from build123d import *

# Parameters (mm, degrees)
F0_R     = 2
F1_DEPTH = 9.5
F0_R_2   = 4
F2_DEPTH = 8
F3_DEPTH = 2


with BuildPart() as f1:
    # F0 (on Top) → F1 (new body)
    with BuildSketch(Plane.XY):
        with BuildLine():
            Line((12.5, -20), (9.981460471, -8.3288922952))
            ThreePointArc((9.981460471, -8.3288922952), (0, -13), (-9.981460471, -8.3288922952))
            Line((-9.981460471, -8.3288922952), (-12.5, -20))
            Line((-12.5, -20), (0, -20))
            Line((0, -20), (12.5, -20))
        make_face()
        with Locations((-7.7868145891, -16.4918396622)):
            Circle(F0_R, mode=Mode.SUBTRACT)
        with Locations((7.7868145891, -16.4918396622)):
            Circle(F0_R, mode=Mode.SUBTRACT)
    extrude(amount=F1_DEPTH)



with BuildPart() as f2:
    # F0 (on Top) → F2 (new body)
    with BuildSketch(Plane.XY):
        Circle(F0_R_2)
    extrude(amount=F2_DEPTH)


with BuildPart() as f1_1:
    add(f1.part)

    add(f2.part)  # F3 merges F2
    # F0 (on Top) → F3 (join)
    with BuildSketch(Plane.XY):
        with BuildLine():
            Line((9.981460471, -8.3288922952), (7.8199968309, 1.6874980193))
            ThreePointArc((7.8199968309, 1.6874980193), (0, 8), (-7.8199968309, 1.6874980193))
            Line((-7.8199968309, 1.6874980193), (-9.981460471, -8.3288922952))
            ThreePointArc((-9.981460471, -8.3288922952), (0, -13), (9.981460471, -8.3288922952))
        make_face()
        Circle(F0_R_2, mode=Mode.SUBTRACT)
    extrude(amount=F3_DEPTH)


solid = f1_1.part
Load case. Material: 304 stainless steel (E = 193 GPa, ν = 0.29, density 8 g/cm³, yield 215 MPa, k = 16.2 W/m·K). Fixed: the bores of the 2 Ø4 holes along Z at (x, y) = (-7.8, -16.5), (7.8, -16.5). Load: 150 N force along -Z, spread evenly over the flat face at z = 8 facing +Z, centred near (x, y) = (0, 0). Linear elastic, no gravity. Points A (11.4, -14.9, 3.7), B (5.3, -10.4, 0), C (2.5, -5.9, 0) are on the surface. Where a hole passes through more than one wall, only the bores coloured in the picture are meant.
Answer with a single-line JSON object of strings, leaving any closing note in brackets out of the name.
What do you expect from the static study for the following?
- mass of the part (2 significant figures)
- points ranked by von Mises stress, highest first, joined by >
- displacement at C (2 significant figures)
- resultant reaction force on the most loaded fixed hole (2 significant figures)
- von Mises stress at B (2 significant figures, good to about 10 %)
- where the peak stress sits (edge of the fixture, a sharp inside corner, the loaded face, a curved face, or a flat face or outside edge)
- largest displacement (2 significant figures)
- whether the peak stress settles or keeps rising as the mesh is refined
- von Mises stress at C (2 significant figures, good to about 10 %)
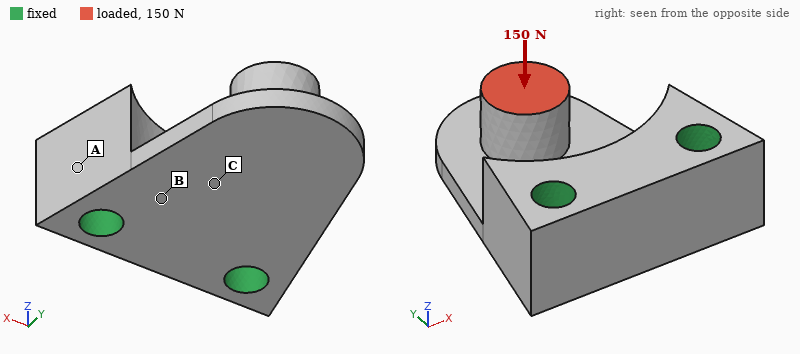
{"mass of the part": "21 g", "points ranked by von Mises stress, highest first, joined by >": "B > C > A", "displacement at C": "13 µm", "resultant reaction force on the most loaded fixed hole": "76 N", "von Mises stress at B": "88 MPa", "where the peak stress sits": "a sharp inside corner", "largest displacement": "67 µm", "whether the peak stress settles or keeps rising as the mesh is refined": "keeps rising", "von Mises stress at C": "67 MPa"}
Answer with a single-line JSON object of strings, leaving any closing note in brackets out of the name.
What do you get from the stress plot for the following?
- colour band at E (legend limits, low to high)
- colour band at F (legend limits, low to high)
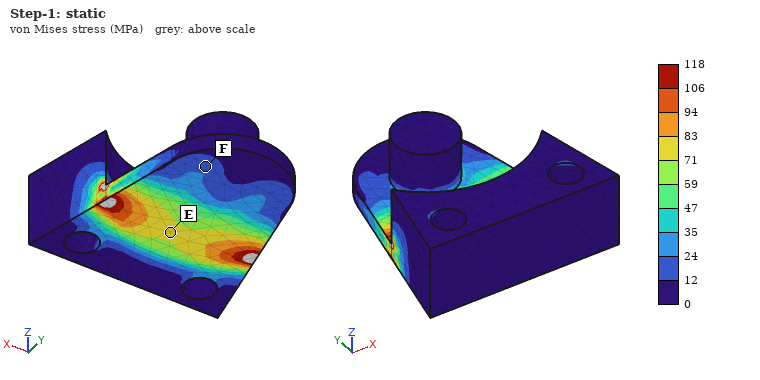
{"colour band at E": "71 to 83 MPa", "colour band at F": "12 to 24 MPa"}
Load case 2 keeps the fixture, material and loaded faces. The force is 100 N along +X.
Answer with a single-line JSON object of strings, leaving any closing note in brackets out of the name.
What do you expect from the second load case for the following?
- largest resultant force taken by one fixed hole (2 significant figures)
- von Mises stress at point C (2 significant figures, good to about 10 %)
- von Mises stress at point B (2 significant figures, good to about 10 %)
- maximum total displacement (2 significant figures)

{"largest resultant force taken by one fixed hole": "110 N", "von Mises stress at point C": "25 MPa", "von Mises stress at point B": "19 MPa", "maximum total displacement": "8.9 µm"}
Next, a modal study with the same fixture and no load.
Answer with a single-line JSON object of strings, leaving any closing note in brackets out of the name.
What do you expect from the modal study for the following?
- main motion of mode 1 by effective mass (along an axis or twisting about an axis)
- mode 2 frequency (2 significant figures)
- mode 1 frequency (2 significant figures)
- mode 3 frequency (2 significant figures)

{"main motion of mode 1 by effective mass": "along Z", "mode 2 frequency": "13 kHz", "mode 1 frequency": "3900 Hz", "mode 3 frequency": "20 kHz"}
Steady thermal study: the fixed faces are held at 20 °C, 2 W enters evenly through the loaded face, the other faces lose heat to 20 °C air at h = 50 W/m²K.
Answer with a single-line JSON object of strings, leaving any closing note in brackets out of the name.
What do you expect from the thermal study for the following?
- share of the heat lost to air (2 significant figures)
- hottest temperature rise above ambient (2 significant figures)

{"share of the heat lost to air": "44 %", "hottest temperature rise above ambient": "42 K"}
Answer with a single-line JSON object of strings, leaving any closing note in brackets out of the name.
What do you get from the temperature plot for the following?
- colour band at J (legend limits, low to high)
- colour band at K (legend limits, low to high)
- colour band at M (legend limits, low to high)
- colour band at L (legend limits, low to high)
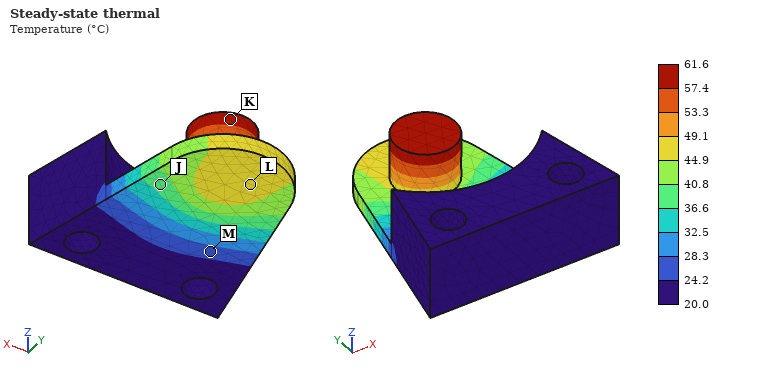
{"colour band at J": "36.6 to 40.8 °C", "colour band at K": "57.4 to 61.6 °C", "colour band at M": "24.2 to 28.3 °C", "colour band at L": "44.9 to 49.1 °C"}
